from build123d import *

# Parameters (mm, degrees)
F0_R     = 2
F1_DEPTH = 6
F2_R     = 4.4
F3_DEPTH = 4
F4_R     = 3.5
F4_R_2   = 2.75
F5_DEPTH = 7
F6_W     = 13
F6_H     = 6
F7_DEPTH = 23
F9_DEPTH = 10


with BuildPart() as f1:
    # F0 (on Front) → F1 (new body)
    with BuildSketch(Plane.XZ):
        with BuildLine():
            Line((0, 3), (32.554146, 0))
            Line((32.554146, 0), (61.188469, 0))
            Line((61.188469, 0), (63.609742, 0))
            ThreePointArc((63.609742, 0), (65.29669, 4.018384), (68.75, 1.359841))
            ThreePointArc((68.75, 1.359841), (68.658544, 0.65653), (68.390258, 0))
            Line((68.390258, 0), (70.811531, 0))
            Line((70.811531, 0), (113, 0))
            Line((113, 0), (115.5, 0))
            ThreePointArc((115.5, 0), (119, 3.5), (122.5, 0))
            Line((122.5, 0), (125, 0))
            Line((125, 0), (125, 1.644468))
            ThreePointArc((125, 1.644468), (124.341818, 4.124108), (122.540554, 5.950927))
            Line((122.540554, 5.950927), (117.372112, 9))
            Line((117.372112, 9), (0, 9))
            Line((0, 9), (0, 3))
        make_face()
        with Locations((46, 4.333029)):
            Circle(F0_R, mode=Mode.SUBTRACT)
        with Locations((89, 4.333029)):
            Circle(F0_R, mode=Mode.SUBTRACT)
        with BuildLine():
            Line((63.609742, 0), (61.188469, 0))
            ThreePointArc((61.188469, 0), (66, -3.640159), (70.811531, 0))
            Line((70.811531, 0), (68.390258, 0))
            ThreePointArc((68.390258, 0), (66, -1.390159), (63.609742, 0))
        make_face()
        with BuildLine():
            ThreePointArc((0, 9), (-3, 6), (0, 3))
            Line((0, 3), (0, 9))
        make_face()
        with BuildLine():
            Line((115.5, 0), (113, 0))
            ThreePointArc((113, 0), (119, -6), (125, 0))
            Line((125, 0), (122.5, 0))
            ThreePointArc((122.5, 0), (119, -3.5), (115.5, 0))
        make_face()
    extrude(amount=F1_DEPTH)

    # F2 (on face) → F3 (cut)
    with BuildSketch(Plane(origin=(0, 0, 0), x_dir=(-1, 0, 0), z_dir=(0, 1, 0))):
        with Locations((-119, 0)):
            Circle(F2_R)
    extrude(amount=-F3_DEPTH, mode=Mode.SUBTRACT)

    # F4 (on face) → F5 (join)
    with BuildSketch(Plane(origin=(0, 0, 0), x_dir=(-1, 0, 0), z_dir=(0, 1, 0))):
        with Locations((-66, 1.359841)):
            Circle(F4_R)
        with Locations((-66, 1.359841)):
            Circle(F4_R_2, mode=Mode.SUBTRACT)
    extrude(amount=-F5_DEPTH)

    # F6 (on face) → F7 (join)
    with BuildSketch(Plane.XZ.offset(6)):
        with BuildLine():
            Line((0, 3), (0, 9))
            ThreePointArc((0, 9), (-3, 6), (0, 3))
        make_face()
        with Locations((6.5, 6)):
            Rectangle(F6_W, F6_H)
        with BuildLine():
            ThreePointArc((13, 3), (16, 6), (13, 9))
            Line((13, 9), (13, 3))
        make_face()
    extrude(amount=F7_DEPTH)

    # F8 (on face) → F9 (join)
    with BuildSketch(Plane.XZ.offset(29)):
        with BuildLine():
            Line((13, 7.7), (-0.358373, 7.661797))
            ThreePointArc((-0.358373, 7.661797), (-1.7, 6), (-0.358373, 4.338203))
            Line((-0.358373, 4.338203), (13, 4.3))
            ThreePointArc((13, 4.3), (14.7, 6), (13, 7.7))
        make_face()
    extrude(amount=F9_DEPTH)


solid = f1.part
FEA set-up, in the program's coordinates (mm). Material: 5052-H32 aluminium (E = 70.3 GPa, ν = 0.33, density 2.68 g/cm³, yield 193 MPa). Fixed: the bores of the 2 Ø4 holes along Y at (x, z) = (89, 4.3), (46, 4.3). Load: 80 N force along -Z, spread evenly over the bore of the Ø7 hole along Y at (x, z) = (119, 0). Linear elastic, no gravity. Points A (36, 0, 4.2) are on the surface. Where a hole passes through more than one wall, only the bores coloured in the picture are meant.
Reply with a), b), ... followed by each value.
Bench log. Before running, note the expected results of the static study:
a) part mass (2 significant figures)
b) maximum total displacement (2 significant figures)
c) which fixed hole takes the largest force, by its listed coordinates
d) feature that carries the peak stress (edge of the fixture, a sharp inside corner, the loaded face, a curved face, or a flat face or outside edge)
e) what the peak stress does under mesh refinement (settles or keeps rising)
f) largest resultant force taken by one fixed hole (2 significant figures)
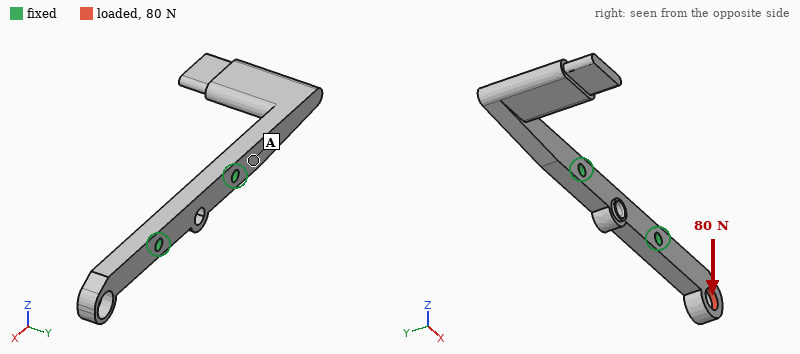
a) 25 g
b) 47 µm
c) (89, 4.3)
d) edge of the fixture
e) keeps rising
f) 90 N
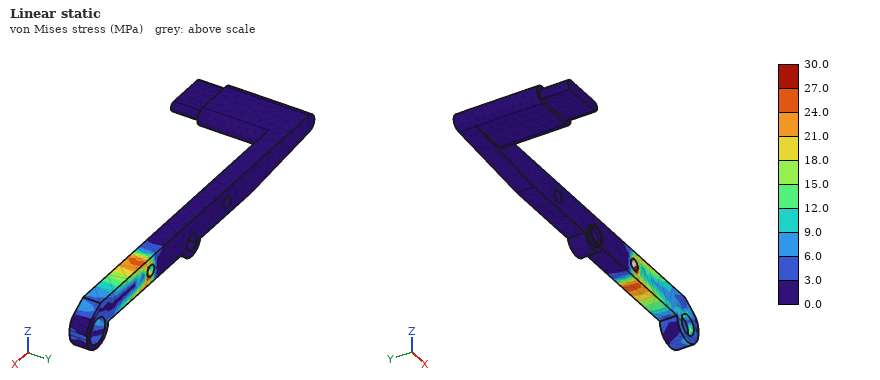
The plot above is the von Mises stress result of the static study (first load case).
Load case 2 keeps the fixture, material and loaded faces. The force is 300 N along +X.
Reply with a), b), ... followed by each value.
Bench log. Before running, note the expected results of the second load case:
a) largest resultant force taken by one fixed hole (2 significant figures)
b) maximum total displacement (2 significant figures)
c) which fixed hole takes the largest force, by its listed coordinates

a) 300 N
b) 56 µm
c) (89, 4.3)
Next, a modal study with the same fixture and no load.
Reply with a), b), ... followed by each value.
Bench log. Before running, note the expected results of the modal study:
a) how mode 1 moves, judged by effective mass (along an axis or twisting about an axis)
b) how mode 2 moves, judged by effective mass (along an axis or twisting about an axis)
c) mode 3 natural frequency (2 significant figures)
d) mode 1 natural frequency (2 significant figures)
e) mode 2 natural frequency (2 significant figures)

a) along Y
b) along Z
c) 3100 Hz
d) 970 Hz
e) 1100 Hz
